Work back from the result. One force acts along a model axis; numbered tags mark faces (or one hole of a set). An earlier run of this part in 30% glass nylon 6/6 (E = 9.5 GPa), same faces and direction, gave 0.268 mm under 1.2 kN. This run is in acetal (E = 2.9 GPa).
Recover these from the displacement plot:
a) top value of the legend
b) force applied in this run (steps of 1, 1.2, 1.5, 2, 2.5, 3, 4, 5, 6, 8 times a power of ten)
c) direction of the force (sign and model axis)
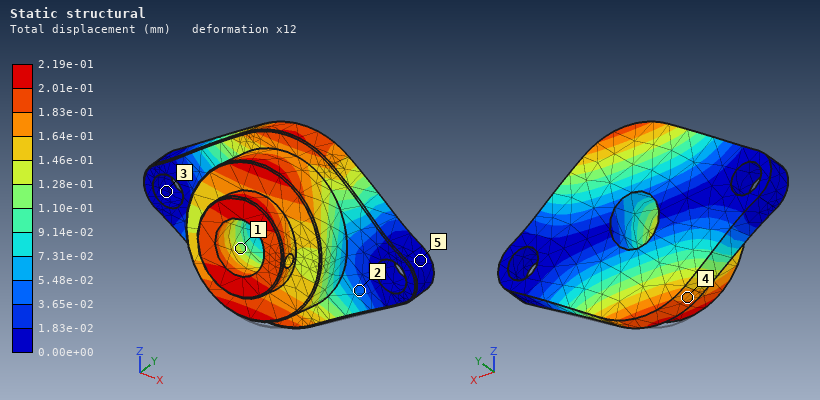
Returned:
2.19e-01 mm
300 N
+Z
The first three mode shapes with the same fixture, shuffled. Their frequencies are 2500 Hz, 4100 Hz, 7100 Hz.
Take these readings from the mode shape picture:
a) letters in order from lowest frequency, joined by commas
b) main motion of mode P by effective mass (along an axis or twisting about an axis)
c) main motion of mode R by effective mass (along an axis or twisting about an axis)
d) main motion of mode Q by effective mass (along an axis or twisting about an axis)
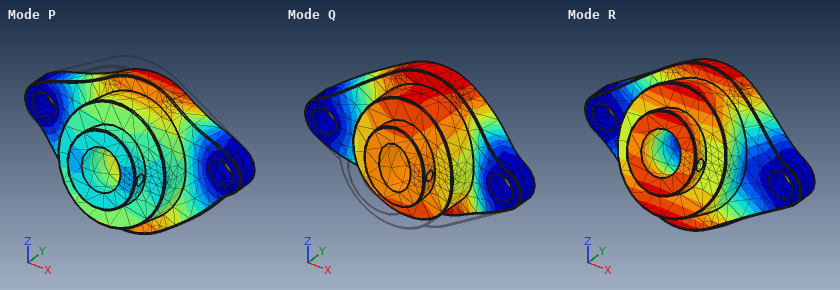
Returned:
R, Q, P
along Z
along Z
along Y
